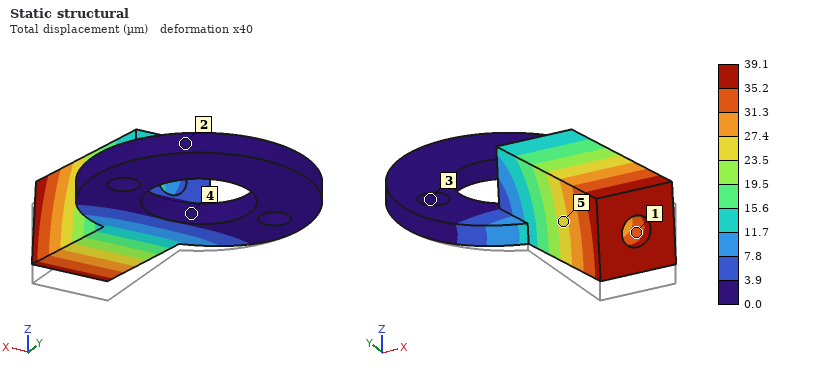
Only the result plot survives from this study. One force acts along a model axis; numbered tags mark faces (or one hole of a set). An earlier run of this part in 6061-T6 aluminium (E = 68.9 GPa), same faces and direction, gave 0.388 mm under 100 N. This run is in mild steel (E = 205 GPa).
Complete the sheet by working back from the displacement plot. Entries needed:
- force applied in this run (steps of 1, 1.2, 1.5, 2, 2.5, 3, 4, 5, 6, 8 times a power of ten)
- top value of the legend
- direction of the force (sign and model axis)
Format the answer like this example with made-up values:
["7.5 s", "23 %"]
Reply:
["30 N", "39.1 µm", "+Z"]
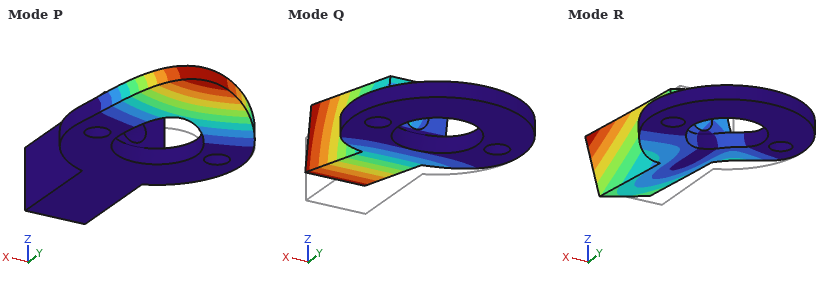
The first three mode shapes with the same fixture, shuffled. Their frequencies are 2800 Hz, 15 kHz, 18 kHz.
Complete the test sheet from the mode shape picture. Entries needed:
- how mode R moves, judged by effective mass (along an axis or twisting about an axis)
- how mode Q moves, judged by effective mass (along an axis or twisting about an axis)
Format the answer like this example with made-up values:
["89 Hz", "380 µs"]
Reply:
["along X", "along Z"]
